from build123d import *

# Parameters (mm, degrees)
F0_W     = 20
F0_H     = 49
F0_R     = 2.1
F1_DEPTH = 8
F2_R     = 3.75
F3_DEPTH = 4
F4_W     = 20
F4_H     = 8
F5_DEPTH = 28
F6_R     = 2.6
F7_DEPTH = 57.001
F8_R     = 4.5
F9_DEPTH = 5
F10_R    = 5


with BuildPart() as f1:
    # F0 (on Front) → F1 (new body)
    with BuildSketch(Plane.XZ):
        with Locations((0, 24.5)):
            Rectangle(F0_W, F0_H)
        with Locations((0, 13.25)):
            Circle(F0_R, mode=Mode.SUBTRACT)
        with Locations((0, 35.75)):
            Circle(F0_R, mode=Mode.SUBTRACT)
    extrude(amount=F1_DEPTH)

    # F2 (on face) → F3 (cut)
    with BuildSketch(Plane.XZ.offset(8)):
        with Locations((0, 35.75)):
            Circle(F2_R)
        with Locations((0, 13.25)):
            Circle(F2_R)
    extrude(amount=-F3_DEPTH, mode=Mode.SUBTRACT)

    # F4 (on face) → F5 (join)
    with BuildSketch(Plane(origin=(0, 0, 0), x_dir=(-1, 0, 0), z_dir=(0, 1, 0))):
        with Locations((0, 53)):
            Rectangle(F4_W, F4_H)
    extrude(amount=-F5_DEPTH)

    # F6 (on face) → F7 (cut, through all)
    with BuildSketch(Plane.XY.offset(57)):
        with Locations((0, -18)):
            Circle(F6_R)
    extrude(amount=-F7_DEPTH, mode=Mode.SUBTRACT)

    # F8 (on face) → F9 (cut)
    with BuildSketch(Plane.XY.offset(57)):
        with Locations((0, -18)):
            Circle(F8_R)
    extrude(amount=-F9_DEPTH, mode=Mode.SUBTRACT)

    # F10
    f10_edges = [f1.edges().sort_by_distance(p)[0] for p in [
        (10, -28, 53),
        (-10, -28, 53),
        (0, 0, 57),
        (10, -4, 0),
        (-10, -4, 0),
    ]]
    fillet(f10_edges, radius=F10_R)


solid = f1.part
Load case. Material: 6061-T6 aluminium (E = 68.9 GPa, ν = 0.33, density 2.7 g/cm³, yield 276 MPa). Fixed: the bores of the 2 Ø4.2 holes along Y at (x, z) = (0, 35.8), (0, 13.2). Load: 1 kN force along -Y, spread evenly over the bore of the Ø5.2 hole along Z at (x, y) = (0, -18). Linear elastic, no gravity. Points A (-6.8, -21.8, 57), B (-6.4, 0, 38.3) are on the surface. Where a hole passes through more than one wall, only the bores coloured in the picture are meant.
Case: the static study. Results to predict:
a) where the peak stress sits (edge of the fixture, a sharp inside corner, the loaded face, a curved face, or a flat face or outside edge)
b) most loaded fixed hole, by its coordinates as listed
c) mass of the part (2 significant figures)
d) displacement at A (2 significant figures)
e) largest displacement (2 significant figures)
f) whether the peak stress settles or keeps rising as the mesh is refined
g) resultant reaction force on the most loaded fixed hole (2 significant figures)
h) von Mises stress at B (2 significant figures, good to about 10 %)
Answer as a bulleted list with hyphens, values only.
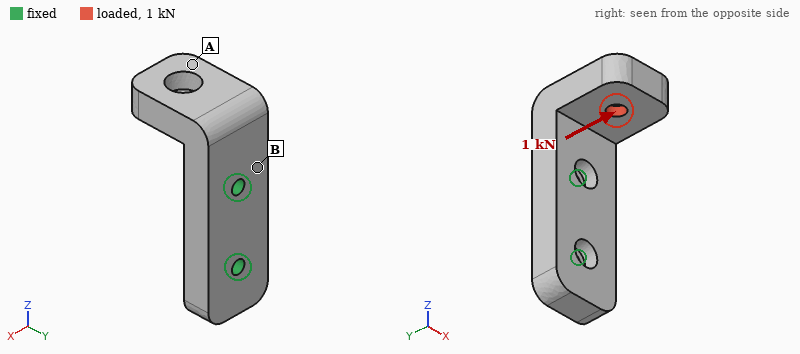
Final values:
- edge of the fixture
- (0, 35.8)
- 30 g
- 83 µm
- 95 µm
- keeps rising
- 1.6 kN
- 49 MPa
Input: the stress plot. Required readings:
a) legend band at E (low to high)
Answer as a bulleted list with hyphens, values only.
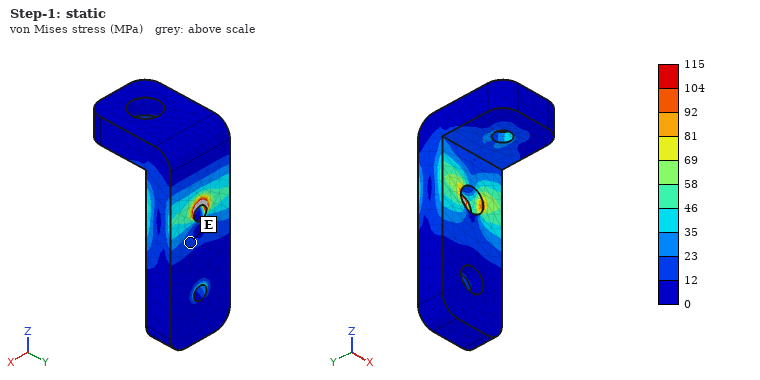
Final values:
- 12 to 23 MPa
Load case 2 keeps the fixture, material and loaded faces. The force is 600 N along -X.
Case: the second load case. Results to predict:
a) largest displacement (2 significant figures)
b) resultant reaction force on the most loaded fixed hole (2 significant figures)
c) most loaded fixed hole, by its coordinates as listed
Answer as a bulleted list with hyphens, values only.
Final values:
- 0.10 mm
- 860 N
- (0, 35.8)
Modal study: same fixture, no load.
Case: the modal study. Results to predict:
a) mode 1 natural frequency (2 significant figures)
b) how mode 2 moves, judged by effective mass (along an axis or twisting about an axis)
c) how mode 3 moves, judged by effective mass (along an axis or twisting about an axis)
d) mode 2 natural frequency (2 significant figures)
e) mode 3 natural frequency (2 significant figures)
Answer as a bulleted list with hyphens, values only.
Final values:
- 4300 Hz
- along X
- along Y
- 4900 Hz
- 12 kHz
